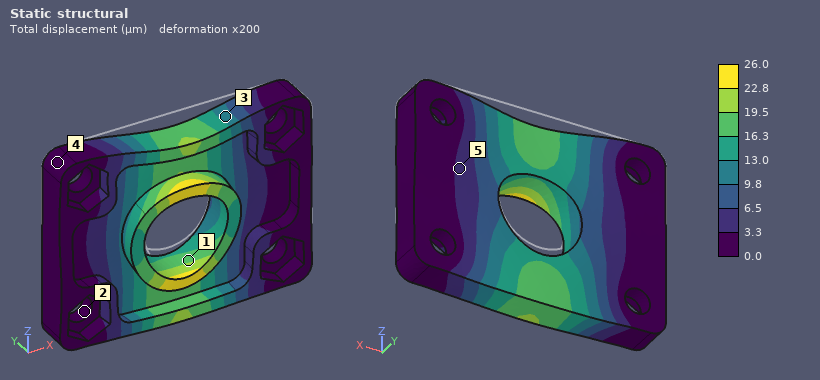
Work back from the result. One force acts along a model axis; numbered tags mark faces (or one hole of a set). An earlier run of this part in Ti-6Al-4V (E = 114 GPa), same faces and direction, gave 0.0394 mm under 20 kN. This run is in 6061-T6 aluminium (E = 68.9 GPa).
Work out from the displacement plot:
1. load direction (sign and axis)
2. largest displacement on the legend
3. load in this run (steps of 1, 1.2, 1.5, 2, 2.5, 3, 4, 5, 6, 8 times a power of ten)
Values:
-Z
26.0 µm
8 kN
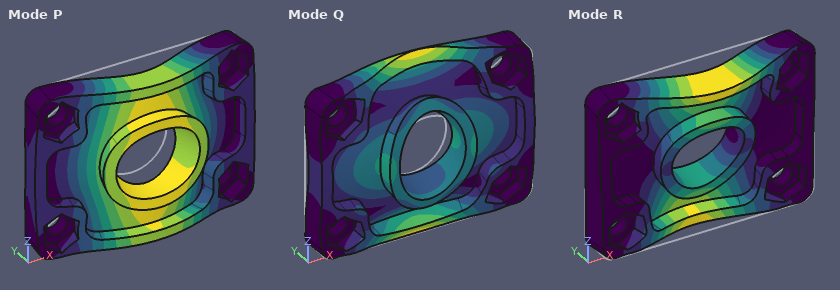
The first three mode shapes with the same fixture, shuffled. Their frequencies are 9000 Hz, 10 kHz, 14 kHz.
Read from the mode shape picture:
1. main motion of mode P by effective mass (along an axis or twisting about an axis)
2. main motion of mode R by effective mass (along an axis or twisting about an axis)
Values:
along Y
twisting about X
